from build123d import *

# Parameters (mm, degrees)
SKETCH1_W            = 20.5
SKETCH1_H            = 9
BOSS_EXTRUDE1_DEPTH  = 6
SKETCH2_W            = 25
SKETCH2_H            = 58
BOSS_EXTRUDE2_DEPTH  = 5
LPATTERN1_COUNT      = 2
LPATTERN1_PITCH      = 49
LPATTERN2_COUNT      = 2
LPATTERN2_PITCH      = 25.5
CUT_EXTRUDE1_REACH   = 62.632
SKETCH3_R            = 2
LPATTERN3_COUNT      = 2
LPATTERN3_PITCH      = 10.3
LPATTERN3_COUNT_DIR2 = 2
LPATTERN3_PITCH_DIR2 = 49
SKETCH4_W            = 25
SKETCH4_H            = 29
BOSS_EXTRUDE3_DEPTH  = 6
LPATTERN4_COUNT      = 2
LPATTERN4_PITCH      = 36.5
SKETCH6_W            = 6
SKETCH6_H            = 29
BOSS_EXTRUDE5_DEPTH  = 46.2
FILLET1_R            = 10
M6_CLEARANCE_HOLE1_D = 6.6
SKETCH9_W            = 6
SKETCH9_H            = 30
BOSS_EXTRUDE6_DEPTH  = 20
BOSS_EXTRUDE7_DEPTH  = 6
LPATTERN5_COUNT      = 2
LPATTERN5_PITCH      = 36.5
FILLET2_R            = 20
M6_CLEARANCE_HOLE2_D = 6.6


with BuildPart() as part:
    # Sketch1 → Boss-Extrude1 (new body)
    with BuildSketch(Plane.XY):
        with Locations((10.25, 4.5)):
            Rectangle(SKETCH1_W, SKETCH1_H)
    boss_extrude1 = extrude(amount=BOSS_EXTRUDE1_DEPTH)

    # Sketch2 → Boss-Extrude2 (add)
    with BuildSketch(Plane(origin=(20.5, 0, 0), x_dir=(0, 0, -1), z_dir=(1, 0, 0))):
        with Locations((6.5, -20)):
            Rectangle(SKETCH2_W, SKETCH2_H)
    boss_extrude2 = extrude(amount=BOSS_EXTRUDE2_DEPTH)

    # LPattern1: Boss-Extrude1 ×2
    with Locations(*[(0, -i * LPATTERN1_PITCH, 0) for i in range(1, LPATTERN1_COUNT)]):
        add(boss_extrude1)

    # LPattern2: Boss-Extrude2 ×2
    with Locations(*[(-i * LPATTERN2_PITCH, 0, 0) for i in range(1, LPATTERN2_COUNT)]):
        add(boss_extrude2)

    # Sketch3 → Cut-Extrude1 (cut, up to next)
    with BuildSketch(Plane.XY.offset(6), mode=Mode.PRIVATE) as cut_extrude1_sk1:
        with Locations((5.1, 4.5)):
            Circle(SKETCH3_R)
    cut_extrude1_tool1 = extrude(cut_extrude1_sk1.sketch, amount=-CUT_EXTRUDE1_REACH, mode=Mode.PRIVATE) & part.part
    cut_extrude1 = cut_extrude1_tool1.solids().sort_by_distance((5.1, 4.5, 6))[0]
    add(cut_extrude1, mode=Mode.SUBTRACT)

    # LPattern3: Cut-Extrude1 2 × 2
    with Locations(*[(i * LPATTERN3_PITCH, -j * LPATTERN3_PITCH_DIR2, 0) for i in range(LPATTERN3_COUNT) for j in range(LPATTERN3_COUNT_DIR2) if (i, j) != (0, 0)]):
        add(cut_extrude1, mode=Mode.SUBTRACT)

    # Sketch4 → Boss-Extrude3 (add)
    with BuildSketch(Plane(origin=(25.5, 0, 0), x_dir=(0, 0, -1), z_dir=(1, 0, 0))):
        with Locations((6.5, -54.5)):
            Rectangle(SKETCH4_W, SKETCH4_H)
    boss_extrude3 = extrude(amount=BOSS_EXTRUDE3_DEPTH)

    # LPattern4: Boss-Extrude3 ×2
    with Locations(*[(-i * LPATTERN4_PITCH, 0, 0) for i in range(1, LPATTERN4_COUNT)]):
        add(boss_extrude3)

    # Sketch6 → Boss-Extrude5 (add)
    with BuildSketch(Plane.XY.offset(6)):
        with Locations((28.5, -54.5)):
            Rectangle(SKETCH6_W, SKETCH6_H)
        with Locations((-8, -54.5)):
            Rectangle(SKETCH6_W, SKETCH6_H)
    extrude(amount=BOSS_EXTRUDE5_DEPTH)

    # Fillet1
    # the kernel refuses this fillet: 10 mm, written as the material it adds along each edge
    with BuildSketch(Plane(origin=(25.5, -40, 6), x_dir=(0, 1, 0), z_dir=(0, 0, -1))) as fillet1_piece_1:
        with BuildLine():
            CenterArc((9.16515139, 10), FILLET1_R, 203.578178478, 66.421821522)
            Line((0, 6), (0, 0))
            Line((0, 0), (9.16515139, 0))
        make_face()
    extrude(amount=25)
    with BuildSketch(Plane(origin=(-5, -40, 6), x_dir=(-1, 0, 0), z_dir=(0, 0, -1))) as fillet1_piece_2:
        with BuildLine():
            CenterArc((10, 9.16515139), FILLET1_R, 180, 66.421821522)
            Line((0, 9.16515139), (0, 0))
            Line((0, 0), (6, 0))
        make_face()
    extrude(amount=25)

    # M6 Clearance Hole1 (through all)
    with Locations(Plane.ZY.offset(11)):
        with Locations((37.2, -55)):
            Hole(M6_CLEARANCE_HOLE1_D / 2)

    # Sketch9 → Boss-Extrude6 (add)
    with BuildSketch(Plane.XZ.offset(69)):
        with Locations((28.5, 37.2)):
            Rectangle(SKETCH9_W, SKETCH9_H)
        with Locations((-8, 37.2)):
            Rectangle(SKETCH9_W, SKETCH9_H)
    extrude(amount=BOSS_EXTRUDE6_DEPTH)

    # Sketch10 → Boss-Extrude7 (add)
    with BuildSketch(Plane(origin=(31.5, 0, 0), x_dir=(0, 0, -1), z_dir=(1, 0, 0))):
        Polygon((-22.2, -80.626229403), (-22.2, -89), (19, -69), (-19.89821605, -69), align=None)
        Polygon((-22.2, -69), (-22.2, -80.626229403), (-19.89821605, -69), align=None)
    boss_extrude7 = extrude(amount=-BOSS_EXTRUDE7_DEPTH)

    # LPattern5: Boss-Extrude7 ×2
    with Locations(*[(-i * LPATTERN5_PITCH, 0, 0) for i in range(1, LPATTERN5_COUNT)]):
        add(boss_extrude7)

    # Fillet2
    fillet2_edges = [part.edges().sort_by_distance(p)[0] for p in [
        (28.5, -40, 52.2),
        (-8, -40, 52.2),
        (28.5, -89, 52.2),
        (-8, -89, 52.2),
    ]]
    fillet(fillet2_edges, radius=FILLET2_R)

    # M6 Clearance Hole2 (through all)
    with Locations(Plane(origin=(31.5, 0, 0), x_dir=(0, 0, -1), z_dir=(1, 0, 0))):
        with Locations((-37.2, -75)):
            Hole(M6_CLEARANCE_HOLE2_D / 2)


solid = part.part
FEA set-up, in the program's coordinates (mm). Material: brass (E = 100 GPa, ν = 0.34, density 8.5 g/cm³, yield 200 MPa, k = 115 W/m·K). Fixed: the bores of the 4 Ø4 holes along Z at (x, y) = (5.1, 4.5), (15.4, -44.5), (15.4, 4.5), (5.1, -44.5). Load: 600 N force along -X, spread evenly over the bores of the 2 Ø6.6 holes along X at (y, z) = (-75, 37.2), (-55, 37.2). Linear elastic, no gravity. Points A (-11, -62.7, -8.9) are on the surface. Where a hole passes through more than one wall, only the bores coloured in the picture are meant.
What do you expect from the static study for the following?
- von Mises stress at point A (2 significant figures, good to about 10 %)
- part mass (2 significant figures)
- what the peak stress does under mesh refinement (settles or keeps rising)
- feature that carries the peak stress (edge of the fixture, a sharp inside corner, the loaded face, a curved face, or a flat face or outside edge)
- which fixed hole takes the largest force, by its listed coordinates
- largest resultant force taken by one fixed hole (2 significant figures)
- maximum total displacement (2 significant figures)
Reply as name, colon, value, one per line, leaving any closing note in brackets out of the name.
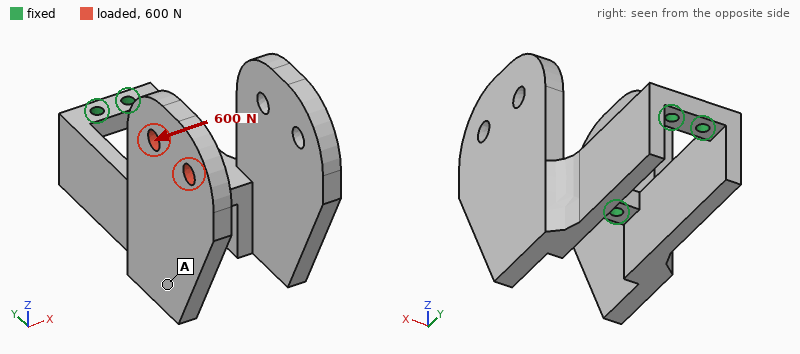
von Mises stress at point A: 46 MPa
part mass: 440 g
what the peak stress does under mesh refinement: keeps rising
feature that carries the peak stress: edge of the fixture
which fixed hole takes the largest force, by its listed coordinates: (5.1, -44.5)
largest resultant force taken by one fixed hole: 790 N
maximum total displacement: 0.71 mm
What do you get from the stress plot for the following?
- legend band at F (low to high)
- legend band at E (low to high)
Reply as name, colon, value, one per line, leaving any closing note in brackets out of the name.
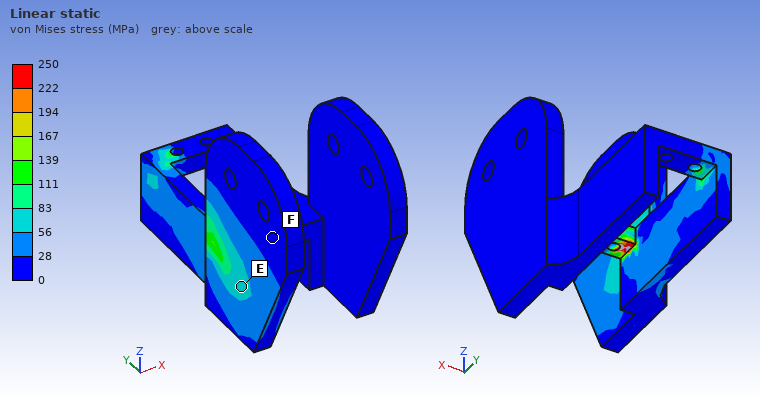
legend band at F: 0 to 28 MPa
legend band at E: 56 to 83 MPa
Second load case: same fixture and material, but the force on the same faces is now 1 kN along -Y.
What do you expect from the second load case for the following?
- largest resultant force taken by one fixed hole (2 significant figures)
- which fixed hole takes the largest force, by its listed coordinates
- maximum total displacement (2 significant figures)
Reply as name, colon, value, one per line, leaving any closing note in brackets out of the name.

largest resultant force taken by one fixed hole: 1.3 kN
which fixed hole takes the largest force, by its listed coordinates: (5.1, -44.5)
maximum total displacement: 0.14 mm
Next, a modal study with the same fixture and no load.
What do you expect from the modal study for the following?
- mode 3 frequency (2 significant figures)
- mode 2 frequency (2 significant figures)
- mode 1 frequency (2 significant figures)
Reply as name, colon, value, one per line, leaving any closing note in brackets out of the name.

mode 3 frequency: 1300 Hz
mode 2 frequency: 660 Hz
mode 1 frequency: 660 Hz
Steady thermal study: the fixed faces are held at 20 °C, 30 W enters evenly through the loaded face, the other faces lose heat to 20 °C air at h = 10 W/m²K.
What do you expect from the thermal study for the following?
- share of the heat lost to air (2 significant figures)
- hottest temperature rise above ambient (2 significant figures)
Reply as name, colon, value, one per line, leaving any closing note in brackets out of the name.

share of the heat lost to air: 13 %
hottest temperature rise above ambient: 74 K
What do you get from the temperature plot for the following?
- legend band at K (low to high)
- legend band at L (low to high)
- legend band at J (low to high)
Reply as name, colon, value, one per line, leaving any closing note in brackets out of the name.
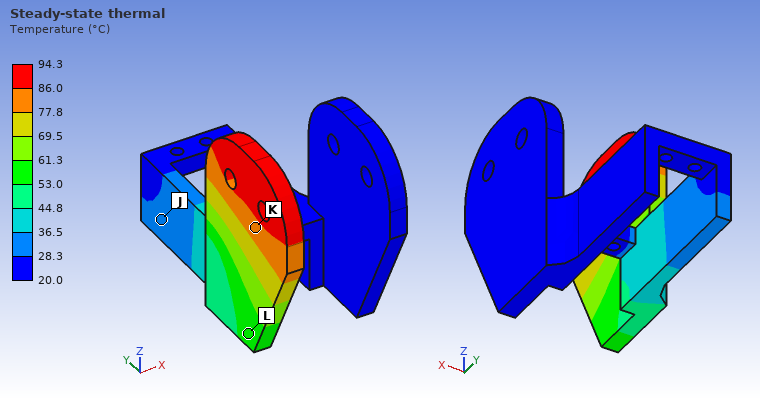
legend band at K: 77.8 to 86.0 °C
legend band at L: 53.0 to 61.3 °C
legend band at J: 28.3 to 36.5 °C
